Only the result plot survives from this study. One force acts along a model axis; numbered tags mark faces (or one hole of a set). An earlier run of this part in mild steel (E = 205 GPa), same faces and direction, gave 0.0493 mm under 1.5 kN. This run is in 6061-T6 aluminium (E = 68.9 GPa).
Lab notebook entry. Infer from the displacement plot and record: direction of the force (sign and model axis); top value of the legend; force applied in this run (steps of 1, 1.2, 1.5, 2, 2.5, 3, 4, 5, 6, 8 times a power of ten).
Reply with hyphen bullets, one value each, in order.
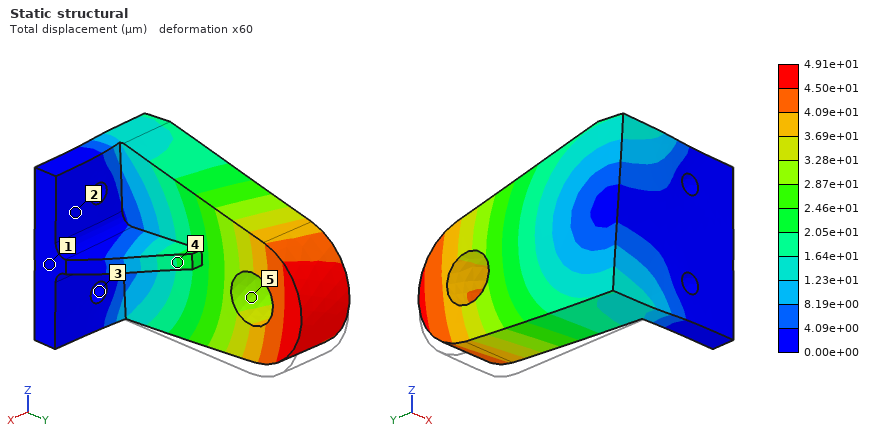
- +Z
- 4.91e+01 µm
- 500 N
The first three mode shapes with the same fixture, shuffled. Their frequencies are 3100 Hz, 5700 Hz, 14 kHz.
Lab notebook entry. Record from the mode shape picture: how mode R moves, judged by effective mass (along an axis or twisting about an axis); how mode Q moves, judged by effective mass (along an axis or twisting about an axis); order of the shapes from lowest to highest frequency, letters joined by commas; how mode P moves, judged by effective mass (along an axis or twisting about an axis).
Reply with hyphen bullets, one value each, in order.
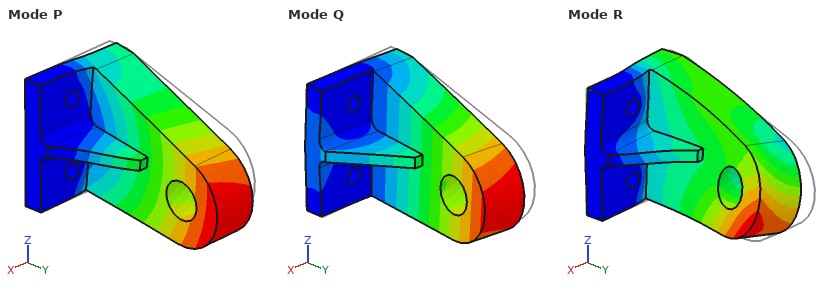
- along Y
- along X
- Q, P, R
- along Z
